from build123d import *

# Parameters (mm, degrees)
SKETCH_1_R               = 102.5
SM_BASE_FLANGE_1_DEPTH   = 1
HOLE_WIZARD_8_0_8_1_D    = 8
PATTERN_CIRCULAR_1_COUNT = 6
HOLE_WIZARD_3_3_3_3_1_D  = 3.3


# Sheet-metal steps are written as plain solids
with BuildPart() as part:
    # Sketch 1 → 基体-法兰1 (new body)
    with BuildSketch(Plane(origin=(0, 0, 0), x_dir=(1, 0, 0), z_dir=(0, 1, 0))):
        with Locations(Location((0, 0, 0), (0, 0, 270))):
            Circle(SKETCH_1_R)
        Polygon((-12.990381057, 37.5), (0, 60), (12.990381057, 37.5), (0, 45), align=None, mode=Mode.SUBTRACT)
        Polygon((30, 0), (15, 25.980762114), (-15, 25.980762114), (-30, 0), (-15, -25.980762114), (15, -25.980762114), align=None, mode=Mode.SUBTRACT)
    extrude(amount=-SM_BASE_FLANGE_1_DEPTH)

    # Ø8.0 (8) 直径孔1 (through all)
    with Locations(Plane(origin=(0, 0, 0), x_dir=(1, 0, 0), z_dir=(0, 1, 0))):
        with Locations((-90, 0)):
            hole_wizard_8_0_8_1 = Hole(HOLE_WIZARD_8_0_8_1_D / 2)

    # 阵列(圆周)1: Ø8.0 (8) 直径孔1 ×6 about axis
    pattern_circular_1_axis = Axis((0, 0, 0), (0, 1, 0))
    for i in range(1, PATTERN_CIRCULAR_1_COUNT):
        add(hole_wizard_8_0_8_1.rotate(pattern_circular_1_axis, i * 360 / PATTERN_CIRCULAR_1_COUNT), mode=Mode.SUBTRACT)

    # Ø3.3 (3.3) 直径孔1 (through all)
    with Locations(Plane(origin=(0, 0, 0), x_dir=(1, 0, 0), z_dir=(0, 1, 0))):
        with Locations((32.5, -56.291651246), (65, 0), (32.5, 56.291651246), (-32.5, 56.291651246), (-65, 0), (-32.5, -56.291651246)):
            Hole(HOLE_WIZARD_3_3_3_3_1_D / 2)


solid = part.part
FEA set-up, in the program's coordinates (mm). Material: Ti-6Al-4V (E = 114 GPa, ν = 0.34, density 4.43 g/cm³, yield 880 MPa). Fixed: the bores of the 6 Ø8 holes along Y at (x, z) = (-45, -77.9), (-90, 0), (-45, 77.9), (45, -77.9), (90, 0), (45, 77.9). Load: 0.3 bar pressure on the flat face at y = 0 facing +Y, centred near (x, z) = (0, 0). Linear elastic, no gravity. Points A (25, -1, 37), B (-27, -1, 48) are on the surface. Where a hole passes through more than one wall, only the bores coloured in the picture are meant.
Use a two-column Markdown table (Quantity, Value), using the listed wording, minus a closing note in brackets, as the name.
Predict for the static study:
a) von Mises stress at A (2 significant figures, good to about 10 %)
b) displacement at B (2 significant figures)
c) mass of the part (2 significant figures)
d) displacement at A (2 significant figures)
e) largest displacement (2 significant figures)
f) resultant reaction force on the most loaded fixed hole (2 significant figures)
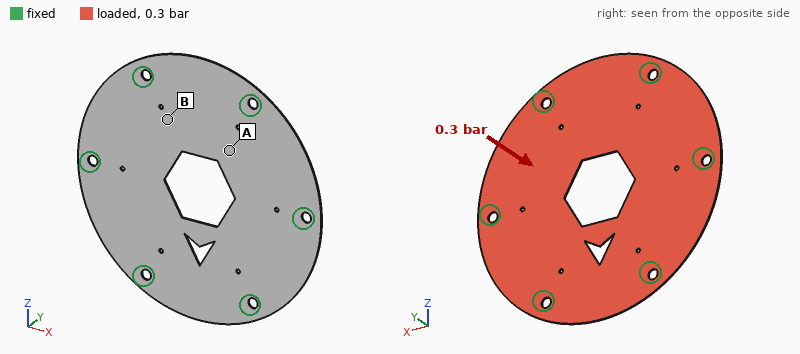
| Quantity | Value |
|---|---|
| von Mises stress at A | 61 MPa |
| displacement at B | 1.5 mm |
| mass of the part | 130 g |
| displacement at A | 2.1 mm |
| largest displacement | 3.2 mm |
| resultant reaction force on the most loaded fixed hole | 150 N |
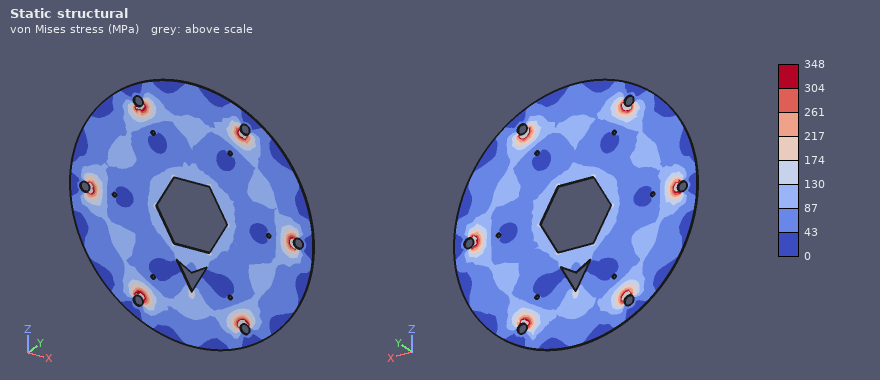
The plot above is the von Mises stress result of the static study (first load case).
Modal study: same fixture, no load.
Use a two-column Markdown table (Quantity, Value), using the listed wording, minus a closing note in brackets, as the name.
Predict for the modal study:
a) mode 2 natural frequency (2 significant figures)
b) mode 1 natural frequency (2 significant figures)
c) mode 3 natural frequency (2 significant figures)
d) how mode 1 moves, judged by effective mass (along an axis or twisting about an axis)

| Quantity | Value |
|---|---|
| mode 2 natural frequency | 510 Hz |
| mode 1 natural frequency | 300 Hz |
| mode 3 natural frequency | 510 Hz |
| how mode 1 moves, judged by effective mass | along Y |
